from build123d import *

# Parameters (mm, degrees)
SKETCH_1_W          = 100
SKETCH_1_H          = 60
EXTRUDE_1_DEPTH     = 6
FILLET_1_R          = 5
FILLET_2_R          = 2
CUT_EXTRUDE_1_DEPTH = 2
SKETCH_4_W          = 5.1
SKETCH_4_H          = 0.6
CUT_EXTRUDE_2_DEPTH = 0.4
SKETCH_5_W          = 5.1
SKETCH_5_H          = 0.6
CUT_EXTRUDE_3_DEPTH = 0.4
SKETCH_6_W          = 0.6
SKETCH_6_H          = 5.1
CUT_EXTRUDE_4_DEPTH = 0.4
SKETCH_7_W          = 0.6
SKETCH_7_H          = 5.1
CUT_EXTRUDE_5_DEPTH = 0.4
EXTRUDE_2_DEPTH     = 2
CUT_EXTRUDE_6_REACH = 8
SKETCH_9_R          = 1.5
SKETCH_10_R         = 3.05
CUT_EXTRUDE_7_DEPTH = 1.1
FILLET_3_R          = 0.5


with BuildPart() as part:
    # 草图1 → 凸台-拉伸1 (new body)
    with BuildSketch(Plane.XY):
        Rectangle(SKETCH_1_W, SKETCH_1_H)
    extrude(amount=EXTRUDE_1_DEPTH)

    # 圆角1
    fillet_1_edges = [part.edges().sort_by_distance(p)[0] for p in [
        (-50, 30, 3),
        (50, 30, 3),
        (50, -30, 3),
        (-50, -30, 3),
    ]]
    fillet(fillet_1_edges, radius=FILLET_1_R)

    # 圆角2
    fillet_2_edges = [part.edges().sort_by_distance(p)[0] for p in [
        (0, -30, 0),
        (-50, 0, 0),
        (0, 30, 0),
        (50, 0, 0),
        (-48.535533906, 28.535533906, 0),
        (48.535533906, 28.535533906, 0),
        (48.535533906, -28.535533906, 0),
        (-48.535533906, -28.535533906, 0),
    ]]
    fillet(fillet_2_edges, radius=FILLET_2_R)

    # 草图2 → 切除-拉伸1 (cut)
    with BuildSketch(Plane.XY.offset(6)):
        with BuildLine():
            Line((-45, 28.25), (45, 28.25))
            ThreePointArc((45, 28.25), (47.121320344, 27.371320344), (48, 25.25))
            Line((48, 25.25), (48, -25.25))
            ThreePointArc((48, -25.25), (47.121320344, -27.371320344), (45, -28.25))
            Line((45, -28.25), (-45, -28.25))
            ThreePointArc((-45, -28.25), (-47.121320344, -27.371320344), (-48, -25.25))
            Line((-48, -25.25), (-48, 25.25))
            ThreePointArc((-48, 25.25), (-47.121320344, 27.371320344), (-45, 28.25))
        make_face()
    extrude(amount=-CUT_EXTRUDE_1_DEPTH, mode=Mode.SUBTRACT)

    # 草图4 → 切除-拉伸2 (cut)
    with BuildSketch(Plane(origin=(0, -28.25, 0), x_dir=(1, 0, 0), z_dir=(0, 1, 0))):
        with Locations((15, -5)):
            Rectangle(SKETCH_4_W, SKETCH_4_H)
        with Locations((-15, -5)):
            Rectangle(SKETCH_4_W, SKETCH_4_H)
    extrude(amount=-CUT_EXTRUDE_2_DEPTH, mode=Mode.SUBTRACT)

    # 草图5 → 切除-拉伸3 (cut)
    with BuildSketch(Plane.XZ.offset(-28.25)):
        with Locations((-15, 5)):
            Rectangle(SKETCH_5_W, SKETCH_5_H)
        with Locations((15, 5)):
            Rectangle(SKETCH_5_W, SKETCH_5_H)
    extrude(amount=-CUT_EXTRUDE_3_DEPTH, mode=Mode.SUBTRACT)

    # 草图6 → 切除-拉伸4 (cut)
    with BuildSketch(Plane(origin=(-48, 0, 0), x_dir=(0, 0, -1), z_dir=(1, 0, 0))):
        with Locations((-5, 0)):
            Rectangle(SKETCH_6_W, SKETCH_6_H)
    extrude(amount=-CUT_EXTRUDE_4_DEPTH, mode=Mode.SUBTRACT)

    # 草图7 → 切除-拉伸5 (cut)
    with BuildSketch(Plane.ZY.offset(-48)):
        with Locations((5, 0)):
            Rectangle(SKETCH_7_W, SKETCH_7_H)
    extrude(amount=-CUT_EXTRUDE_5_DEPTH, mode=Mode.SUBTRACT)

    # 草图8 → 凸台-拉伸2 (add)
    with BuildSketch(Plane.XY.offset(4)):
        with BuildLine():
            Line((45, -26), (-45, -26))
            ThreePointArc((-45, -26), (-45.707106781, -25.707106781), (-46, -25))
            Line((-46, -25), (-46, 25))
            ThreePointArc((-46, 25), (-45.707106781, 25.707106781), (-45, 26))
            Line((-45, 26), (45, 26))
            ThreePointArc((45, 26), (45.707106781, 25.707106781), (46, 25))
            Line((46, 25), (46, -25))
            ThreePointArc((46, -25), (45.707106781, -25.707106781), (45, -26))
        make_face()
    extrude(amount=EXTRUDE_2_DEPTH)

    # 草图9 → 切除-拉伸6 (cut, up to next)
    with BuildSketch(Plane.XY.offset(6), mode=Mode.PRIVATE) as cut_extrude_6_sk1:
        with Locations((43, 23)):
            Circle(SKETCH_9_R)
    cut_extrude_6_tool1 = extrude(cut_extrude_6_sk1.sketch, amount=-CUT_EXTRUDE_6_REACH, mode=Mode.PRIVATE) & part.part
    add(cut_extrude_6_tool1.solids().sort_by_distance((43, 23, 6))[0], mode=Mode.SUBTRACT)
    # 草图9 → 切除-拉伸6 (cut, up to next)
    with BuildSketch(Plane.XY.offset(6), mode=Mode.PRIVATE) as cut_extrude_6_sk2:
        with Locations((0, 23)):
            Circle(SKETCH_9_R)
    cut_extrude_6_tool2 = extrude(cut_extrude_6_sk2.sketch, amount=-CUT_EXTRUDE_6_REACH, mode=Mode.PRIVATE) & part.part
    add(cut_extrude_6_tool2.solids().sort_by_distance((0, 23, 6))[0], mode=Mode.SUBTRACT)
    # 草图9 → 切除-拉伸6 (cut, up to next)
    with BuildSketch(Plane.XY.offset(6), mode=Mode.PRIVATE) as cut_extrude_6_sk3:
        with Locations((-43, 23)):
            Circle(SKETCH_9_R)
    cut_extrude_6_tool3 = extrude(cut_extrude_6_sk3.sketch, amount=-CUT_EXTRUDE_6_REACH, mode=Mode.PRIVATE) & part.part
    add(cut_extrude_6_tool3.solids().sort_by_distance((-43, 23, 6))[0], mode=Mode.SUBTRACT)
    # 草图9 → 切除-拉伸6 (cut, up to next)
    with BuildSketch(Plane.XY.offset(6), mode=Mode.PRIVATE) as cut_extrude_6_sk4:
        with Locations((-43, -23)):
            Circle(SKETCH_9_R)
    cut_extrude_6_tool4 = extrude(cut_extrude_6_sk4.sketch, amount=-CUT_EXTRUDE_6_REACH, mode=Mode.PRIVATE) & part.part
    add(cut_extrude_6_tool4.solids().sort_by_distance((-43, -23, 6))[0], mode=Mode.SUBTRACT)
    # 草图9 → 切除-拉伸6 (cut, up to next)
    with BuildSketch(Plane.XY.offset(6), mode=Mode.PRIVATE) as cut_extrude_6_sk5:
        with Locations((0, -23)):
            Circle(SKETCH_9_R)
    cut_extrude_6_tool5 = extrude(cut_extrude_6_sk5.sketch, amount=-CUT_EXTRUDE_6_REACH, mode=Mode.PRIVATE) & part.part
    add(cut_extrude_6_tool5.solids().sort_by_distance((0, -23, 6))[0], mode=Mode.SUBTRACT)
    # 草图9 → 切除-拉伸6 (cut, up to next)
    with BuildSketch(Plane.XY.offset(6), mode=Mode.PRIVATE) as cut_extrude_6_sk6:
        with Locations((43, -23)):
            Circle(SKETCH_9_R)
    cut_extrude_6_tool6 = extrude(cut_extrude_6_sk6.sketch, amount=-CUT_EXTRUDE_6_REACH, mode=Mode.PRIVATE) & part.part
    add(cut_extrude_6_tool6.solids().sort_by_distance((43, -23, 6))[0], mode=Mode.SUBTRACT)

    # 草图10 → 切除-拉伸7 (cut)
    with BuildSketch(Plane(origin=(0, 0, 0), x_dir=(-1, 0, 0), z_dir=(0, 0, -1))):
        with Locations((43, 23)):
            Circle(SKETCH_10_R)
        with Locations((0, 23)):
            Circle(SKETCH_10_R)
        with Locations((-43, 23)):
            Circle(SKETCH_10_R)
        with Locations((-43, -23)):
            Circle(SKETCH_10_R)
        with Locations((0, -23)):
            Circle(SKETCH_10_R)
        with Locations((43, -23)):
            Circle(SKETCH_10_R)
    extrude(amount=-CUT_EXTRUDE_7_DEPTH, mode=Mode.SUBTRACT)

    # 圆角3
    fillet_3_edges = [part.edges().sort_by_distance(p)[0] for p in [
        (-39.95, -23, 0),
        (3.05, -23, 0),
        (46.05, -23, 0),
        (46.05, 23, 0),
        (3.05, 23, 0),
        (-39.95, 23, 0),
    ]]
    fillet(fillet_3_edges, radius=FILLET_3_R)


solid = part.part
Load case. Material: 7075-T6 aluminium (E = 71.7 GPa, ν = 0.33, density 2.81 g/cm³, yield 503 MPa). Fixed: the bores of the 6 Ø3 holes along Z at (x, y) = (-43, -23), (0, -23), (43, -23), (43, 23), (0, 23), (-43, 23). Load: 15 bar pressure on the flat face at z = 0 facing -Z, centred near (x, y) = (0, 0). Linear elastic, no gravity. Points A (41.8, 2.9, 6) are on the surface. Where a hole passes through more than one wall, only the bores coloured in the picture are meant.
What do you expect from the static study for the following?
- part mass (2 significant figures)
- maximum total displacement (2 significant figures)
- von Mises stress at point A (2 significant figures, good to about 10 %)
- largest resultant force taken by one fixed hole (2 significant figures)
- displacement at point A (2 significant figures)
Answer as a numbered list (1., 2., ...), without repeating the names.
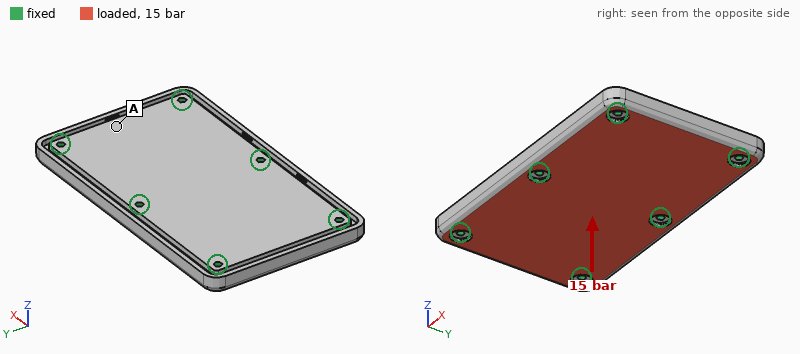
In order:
1. 95 g
2. 43 µm
3. 29 MPa
4. 1.9 kN
5. 29 µm
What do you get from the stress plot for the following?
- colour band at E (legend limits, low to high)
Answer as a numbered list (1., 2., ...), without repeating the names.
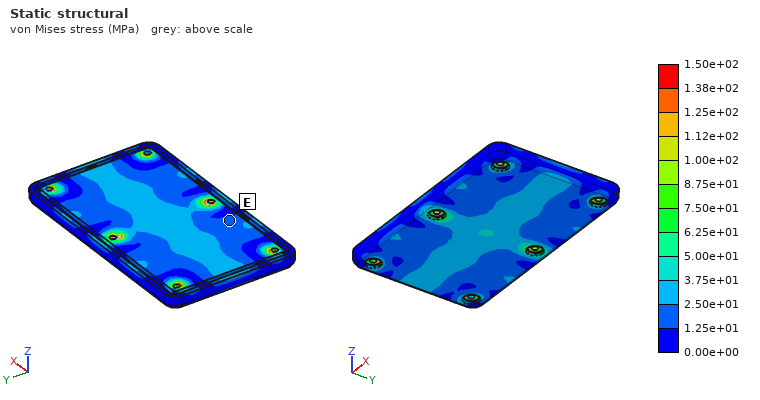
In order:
1. 1.25e+01 to 2.50e+01 MPa
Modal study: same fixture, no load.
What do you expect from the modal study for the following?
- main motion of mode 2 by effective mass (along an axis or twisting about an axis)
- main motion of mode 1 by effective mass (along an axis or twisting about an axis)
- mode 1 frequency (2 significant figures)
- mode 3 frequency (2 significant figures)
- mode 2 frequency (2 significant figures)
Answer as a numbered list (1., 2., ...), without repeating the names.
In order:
1. twisting about Y
2. along Z
3. 8400 Hz
4. 13 kHz
5. 9100 Hz
